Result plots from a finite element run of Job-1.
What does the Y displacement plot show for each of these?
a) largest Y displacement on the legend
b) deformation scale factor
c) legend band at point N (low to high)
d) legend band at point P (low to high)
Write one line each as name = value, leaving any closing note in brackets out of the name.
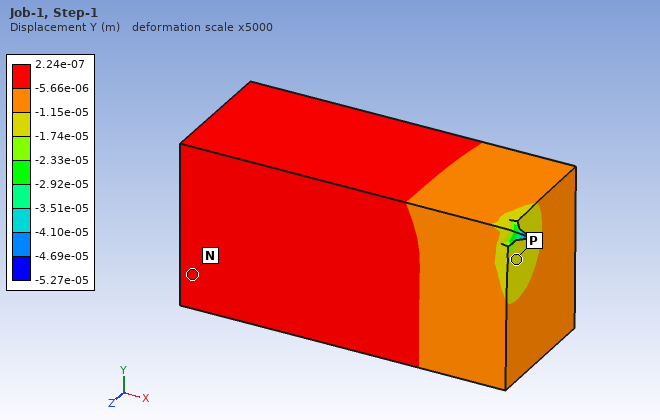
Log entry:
largest Y displacement on the legend = 2.24e-07 m
deformation scale factor = 5000
legend band at point N = -5.66e-06 to 2.24e-07 m
legend band at point P = -1.74e-05 to -1.15e-05 m
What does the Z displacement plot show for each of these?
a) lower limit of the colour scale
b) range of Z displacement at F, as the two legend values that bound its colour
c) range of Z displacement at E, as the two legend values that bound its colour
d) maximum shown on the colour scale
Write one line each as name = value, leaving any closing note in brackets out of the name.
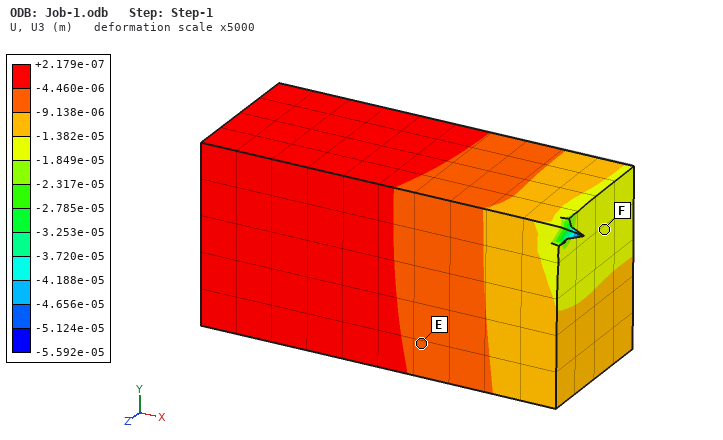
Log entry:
lower limit of the colour scale = -5.592e-05 m
range of Z displacement at F, as the two legend values that bound its colour = -1.849e-05 to -1.382e-05 m
range of Z displacement at E, as the two legend values that bound its colour = -9.138e-06 to -4.460e-06 m
maximum shown on the colour scale = +2.179e-07 m
